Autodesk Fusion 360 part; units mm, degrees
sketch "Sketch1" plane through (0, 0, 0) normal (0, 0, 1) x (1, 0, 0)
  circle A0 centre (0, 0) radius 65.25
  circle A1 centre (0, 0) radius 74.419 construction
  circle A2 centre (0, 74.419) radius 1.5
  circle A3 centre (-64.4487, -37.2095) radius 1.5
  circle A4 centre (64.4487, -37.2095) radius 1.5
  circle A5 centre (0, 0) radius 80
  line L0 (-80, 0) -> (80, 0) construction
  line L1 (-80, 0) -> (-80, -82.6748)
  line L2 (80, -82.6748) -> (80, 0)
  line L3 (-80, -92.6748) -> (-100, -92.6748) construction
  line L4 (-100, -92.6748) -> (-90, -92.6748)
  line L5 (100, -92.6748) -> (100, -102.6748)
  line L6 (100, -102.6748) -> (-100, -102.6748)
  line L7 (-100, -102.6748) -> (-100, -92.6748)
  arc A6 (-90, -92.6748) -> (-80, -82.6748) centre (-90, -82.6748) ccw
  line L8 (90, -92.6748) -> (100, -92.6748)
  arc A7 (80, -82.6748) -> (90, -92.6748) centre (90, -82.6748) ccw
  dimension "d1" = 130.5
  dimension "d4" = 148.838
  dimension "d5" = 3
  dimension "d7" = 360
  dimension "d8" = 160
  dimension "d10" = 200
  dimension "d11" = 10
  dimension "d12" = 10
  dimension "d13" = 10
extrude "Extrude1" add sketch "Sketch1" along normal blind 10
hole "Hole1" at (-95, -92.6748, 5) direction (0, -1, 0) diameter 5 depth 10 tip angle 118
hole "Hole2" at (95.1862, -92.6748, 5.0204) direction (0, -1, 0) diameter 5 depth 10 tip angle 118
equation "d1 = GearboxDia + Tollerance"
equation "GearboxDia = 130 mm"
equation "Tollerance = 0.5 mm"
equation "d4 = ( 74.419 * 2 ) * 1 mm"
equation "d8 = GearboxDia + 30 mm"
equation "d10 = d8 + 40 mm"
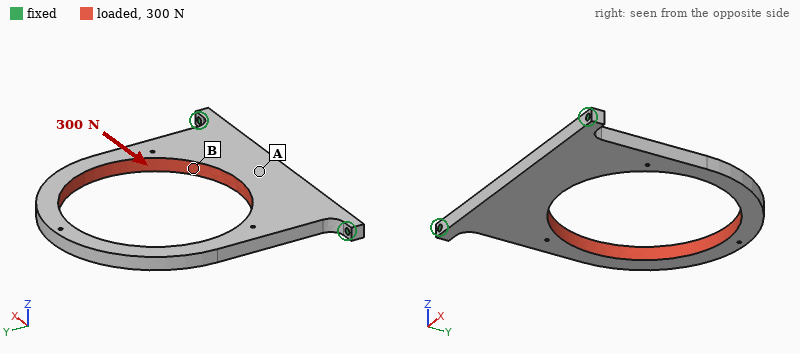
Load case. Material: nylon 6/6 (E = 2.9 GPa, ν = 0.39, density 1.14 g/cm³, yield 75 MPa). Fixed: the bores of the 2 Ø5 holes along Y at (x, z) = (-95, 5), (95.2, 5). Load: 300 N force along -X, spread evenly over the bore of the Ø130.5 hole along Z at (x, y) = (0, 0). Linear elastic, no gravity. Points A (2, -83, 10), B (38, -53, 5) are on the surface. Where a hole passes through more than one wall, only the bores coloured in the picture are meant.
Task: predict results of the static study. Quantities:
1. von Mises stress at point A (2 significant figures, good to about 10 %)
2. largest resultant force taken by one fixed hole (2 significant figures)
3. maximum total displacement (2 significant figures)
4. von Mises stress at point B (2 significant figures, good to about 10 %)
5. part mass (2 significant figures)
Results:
0.88 MPa
220 N
0.76 mm
2.5 MPa
150 g
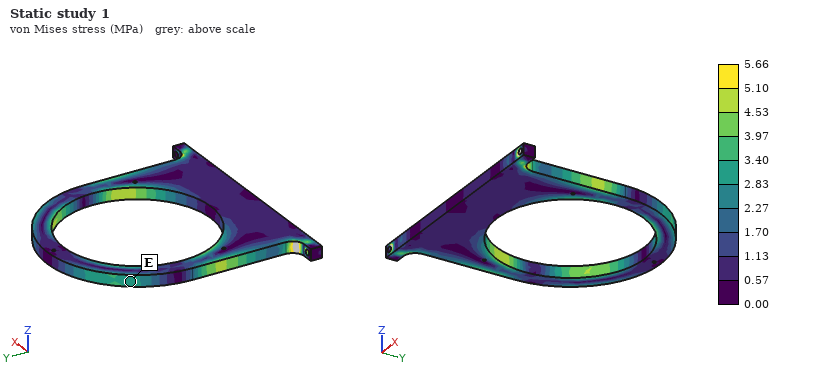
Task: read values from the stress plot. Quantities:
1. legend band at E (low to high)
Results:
2.83 to 3.40 MPa
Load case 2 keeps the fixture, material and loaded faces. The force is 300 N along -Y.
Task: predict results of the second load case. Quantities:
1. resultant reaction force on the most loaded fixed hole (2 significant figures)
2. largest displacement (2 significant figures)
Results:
180 N
0.14 mm
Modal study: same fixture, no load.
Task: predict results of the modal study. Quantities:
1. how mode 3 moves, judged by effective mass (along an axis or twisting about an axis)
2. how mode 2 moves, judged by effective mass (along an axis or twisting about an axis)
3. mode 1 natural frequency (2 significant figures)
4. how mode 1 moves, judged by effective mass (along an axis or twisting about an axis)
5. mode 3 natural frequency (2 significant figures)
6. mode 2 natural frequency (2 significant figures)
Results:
along Z
twisting about Y
58 Hz
along Z
280 Hz
200 Hz
